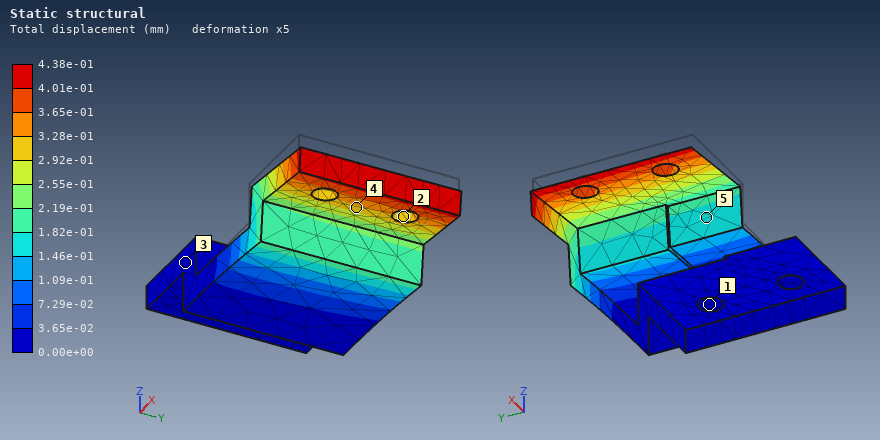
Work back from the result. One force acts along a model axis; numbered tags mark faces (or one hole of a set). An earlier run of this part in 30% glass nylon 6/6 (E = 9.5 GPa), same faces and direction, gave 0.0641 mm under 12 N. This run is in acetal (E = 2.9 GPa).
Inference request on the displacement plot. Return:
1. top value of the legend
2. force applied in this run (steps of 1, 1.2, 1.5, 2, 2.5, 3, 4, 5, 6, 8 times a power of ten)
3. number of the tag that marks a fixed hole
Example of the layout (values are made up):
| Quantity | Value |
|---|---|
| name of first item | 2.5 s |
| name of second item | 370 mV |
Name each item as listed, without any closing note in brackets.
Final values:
| Quantity | Value |
|---|---|
| top value of the legend | 4.38e-01 mm |
| force applied in this run | 25 N |
| number of the tag that marks a fixed hole | 1 |
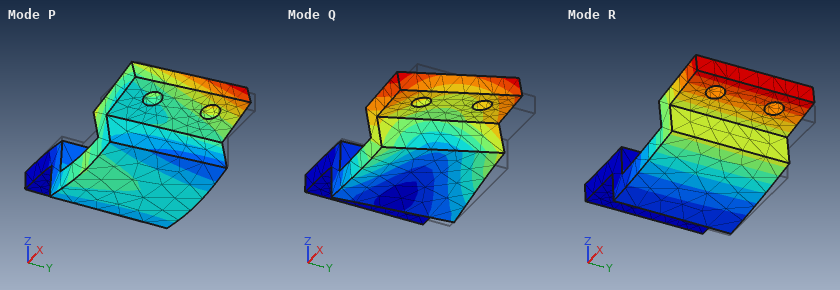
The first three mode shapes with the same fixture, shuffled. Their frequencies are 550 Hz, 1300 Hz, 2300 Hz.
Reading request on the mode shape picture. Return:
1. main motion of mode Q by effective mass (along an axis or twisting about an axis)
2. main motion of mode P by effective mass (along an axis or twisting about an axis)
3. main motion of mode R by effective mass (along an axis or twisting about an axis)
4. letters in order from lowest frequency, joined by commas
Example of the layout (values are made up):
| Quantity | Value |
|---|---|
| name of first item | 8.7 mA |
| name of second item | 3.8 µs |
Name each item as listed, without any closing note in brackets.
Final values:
| Quantity | Value |
|---|---|
| main motion of mode Q by effective mass | along Y |
| main motion of mode P by effective mass | along X |
| main motion of mode R by effective mass | along Z |
| letters in order from lowest frequency, joined by commas | R, Q, P |
